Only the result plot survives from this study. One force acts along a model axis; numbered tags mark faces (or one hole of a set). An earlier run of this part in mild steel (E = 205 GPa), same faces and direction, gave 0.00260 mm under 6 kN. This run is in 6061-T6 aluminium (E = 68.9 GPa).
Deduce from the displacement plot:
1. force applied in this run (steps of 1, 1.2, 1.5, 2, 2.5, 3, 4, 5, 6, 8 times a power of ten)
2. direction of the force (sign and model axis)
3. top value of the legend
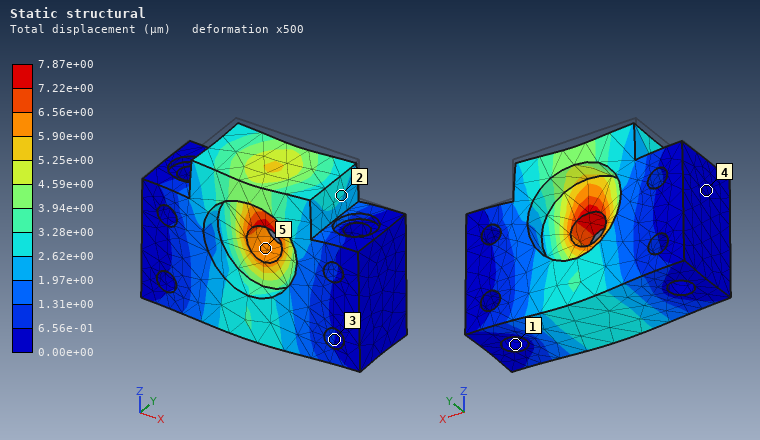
6 kN
-Z
7.87e+00 µm
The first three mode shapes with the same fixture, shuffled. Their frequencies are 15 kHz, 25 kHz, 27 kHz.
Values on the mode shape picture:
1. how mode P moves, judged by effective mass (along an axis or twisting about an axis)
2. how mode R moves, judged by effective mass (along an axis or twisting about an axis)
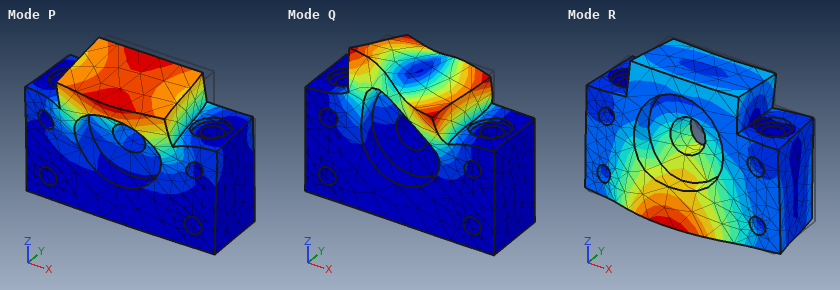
along Y
along Y
